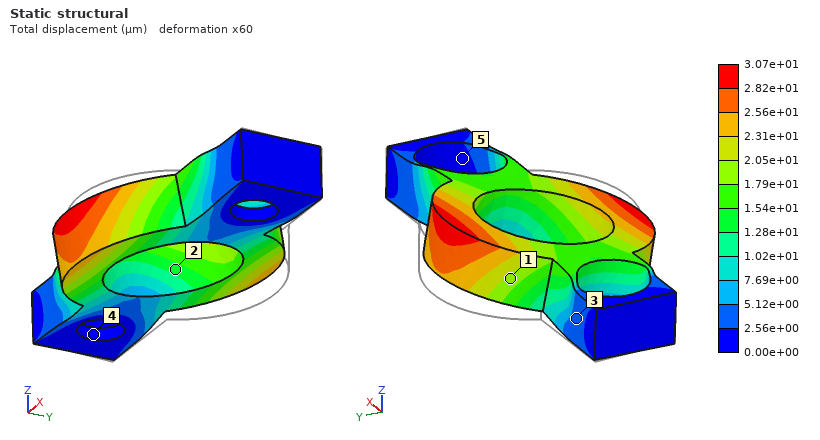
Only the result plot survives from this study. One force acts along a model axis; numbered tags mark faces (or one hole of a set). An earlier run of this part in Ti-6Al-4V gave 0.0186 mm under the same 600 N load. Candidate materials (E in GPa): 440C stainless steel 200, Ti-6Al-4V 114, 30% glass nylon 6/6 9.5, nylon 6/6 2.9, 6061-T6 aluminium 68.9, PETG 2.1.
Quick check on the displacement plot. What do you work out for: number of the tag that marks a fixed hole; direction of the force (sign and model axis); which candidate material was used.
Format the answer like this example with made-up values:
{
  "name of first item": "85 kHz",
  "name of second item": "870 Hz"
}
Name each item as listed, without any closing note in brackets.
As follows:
{
  "number of the tag that marks a fixed hole": "4",
  "direction of the force": "-Y",
  "which candidate material was used": "6061-T6 aluminium"
}
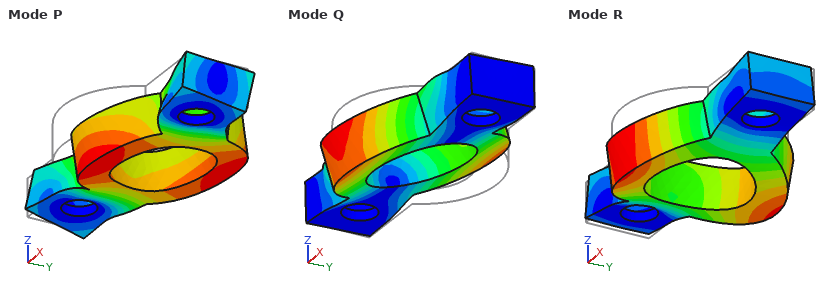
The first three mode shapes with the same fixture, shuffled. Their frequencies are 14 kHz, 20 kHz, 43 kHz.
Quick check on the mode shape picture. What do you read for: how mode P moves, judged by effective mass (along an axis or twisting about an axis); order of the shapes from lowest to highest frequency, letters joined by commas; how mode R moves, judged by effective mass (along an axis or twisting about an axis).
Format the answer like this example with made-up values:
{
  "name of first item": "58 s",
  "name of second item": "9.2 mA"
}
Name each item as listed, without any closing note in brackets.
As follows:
{
  "how mode P moves, judged by effective mass": "along Y",
  "order of the shapes from lowest to highest frequency, letters joined by commas": "Q, R, P",
  "how mode R moves, judged by effective mass": "along Z"
}
